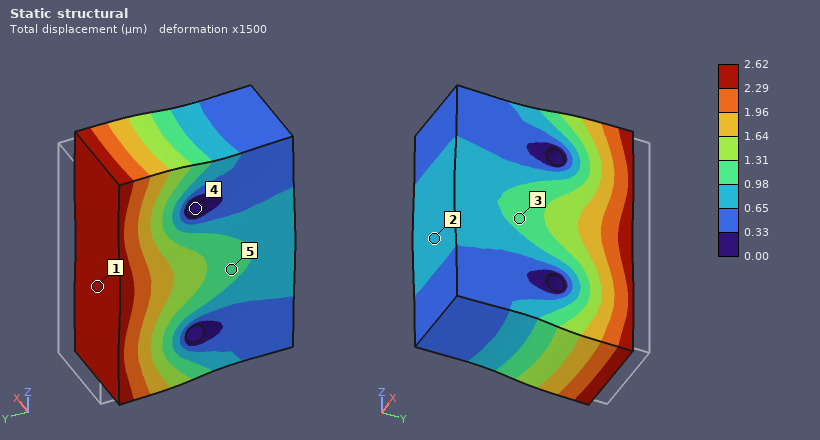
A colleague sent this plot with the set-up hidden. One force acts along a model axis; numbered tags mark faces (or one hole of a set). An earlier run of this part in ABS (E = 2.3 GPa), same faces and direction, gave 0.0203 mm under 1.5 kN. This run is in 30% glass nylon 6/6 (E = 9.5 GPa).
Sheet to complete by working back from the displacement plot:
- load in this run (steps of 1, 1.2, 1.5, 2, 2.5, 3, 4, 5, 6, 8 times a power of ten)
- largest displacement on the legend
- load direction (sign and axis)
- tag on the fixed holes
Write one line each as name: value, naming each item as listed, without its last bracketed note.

load in this run: 800 N
largest displacement on the legend: 2.62 µm
load direction: -Y
tag on the fixed holes: 4
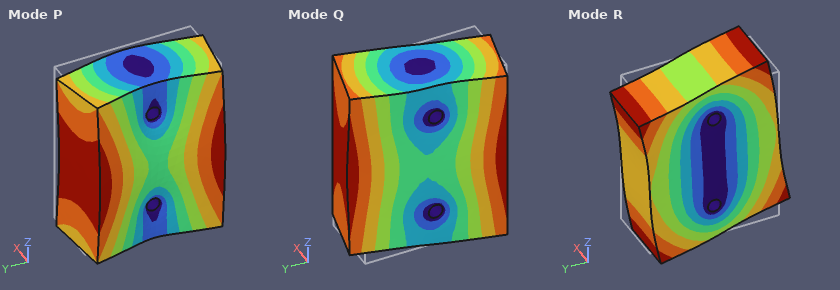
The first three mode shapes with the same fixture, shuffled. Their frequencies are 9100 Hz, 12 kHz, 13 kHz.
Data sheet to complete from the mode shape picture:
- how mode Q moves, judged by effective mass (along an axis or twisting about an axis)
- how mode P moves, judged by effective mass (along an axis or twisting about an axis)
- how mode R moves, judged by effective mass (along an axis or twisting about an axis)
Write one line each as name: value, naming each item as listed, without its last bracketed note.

how mode Q moves, judged by effective mass: twisting about Z
how mode P moves, judged by effective mass: along X
how mode R moves, judged by effective mass: twisting about X
